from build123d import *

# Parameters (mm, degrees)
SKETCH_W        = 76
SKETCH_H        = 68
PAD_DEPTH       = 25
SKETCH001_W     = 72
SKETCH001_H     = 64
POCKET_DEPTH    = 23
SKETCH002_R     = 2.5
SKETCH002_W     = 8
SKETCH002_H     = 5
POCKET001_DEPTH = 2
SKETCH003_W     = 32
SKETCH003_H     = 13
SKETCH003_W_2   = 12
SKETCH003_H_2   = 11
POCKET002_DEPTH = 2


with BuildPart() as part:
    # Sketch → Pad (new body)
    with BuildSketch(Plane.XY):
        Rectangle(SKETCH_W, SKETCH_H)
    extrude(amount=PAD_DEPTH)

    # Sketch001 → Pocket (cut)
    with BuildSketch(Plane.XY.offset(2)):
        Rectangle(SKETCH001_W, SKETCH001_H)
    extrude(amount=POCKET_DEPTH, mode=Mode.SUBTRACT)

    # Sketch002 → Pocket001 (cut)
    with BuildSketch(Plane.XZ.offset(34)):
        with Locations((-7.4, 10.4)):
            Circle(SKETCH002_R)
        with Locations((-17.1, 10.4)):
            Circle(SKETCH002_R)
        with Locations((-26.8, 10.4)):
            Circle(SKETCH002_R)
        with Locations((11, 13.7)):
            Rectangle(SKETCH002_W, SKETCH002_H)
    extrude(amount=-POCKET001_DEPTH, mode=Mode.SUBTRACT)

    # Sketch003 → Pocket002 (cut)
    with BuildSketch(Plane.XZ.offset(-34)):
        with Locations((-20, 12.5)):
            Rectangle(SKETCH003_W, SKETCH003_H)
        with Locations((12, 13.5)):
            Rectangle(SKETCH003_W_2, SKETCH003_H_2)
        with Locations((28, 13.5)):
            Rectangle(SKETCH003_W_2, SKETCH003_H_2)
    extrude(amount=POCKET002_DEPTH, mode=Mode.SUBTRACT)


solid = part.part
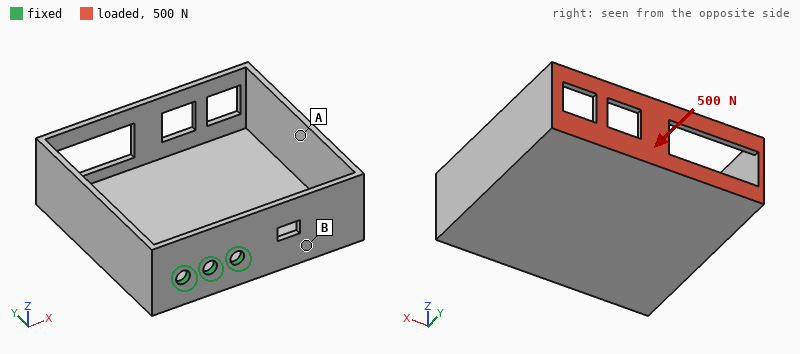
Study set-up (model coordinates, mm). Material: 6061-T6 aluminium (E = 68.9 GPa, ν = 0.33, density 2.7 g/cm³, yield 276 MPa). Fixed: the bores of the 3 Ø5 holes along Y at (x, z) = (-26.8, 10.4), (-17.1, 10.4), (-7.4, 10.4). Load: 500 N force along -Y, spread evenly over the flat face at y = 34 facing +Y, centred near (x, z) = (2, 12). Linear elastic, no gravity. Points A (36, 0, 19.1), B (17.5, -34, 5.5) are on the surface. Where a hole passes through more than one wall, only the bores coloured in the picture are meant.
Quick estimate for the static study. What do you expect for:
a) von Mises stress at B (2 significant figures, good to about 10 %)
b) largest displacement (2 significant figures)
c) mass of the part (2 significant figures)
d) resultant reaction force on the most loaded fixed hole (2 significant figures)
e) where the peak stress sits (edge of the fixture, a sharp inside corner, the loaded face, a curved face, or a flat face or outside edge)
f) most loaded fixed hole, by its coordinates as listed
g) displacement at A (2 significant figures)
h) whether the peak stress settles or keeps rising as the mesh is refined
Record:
54 MPa
1.2 mm
58 g
620 N
edge of the fixture
(-7.4, 10.4)
0.71 mm
keeps rising
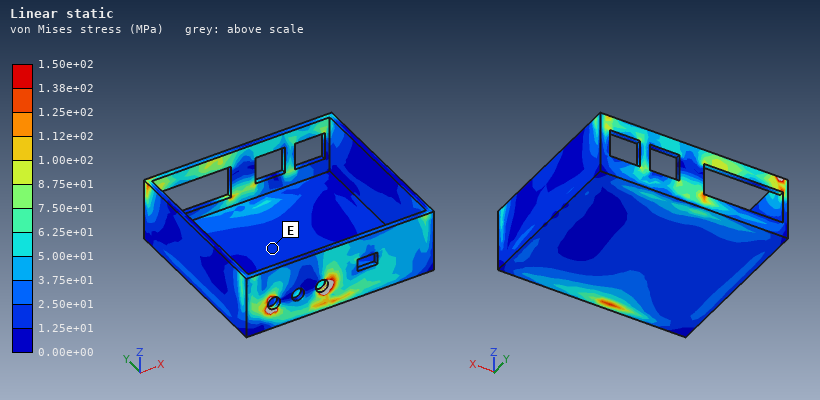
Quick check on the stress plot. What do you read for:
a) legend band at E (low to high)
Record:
1.25e+01 to 2.50e+01 MPa
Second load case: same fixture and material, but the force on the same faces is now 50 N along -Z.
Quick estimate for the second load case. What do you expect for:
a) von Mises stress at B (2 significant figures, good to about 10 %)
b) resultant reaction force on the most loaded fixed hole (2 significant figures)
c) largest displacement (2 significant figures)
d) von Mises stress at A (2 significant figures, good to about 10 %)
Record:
25 MPa
90 N
0.86 mm
11 MPa
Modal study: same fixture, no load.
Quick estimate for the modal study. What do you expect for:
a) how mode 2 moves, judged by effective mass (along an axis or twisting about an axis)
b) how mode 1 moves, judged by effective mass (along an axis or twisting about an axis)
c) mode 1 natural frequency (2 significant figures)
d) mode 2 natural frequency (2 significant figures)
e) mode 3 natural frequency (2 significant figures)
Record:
along X
along Z
310 Hz
560 Hz
960 Hz
